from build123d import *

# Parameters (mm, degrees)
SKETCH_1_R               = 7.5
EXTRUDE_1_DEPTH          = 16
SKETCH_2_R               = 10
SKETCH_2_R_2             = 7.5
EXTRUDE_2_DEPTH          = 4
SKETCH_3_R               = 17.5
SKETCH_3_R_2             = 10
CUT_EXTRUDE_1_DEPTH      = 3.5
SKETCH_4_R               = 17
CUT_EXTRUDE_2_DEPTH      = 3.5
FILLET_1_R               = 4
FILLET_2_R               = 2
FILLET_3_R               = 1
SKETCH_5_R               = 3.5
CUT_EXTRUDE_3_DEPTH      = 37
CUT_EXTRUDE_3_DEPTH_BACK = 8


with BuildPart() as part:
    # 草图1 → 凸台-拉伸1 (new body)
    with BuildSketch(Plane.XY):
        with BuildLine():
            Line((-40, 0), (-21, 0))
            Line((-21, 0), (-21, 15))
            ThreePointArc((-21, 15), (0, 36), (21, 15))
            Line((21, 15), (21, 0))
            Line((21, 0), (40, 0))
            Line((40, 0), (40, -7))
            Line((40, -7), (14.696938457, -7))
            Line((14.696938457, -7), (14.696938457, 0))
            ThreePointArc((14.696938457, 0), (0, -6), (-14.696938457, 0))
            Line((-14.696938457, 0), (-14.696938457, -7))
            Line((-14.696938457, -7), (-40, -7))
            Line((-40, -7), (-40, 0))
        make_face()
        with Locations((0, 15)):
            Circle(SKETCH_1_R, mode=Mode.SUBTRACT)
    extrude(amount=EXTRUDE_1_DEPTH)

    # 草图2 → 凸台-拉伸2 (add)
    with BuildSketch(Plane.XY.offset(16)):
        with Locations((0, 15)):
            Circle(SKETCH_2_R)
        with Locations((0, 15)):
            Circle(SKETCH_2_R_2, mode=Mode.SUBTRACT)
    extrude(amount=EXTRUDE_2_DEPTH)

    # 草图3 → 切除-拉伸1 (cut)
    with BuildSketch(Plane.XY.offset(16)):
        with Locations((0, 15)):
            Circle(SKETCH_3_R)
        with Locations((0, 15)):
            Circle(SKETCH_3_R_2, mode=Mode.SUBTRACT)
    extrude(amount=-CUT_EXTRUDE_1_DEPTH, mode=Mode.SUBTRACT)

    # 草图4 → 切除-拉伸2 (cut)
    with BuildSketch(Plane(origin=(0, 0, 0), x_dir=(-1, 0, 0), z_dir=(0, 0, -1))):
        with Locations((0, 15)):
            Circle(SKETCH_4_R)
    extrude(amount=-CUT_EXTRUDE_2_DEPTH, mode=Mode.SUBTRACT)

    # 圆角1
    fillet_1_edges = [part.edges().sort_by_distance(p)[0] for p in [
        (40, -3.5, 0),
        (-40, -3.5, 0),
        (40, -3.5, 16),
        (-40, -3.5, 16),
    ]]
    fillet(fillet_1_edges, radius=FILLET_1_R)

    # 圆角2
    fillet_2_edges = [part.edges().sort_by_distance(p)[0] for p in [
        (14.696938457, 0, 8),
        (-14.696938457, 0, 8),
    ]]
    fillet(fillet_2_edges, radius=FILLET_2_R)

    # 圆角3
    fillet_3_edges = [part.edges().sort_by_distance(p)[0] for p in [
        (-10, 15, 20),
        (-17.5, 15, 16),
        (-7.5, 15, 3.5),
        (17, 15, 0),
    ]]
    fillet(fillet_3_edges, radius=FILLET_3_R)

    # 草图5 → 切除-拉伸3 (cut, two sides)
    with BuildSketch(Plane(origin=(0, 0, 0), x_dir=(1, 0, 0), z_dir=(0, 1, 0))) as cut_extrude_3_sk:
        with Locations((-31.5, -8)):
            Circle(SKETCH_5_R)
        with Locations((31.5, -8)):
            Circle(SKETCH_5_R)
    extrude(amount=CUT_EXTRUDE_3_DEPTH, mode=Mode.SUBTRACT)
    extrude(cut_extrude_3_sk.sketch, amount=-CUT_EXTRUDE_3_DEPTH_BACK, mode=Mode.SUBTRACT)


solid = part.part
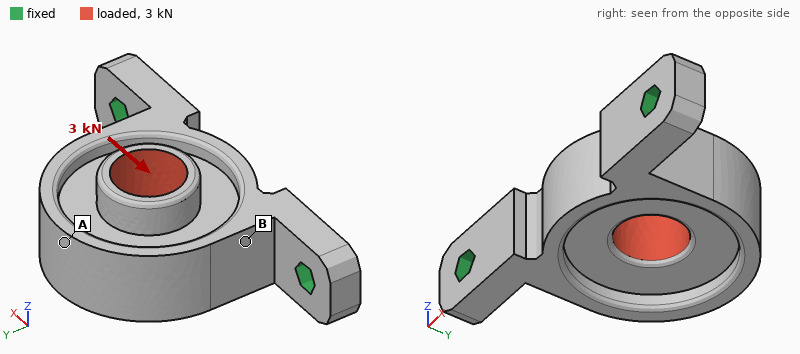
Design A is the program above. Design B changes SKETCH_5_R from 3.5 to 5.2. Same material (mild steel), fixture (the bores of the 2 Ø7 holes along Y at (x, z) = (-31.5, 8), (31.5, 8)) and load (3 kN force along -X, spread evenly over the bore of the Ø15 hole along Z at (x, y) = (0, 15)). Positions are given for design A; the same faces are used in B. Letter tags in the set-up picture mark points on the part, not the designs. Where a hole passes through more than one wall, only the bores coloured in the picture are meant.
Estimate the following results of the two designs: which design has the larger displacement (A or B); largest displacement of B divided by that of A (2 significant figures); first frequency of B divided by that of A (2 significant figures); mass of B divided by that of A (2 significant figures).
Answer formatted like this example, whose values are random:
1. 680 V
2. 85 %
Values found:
1. A
2. 0.92
3. 1.1
4. 0.97
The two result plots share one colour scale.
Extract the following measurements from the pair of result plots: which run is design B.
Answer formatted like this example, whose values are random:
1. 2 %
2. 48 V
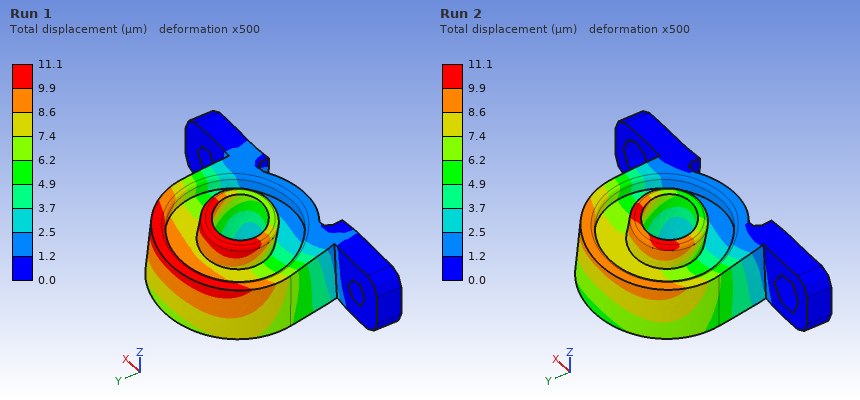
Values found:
1. Run 2
